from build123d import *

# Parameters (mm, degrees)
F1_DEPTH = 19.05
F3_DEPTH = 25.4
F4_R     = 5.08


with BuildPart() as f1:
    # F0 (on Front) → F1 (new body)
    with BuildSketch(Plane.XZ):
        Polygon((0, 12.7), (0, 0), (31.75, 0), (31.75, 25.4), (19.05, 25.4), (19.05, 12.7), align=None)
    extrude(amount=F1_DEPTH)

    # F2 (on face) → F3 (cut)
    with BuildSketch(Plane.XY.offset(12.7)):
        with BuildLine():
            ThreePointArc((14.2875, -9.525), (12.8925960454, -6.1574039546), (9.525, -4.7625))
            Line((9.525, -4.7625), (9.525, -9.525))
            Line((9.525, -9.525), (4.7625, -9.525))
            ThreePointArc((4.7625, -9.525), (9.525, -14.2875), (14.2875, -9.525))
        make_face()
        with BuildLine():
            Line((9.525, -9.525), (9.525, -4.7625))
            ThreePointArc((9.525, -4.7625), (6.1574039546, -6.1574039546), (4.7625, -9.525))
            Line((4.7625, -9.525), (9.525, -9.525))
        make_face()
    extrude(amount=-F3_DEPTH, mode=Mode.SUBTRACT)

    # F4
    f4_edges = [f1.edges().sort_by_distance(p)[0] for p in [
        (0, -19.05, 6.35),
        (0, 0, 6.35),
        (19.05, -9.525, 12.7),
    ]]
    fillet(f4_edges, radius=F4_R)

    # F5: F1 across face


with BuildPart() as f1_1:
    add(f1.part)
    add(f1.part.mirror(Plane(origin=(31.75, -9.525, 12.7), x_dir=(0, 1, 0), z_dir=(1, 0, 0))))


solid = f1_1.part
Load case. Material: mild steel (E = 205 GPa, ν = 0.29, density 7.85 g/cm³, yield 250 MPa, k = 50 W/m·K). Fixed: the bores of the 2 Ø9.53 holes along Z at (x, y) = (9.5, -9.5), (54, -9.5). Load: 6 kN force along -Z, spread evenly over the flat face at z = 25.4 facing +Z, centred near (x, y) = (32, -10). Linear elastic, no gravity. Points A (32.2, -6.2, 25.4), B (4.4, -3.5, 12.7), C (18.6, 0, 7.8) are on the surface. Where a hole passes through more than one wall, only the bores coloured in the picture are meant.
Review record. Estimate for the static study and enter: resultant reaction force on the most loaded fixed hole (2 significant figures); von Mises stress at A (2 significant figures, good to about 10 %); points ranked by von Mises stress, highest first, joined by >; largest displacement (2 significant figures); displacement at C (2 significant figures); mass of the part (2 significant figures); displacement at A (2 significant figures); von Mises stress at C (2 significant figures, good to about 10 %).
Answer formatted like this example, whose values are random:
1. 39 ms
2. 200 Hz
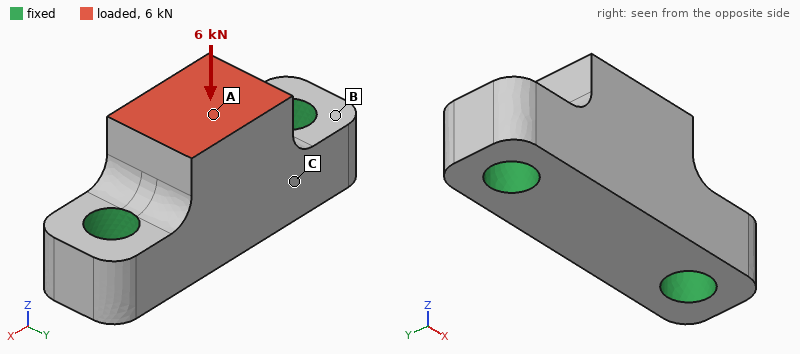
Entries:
1. 3.2 kN
2. 11 MPa
3. C > A > B
4. 2.9 µm
5. 1.4 µm
6. 150 g
7. 2.9 µm
8. 19 MPa
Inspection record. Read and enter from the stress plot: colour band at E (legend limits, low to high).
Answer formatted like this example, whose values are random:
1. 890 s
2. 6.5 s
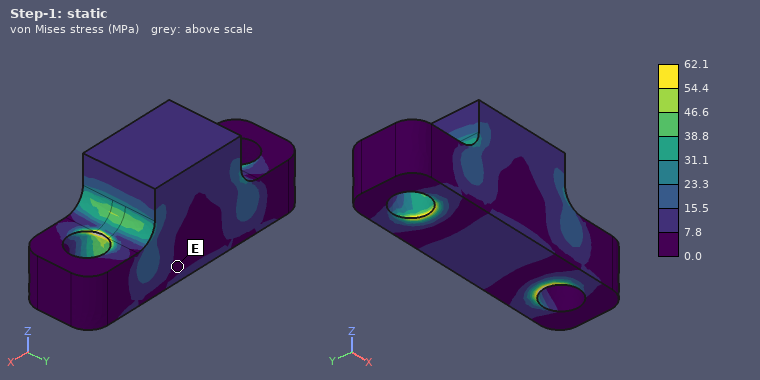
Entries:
1. 0.0 to 7.8 MPa
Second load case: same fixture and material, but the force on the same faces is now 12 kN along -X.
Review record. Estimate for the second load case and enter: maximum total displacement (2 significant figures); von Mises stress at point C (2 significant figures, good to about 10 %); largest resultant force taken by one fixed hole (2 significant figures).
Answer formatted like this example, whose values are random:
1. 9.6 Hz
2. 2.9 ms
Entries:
1. 12 µm
2. 29 MPa
3. 8.6 kN
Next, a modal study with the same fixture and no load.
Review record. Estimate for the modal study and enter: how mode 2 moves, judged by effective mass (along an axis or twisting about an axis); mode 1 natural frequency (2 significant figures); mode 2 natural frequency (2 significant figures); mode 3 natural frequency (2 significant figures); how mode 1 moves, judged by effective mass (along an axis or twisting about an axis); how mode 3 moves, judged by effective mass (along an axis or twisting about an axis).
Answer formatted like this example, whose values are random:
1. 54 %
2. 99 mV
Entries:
1. along Z
2. 16 kHz
3. 26 kHz
4. 31 kHz
5. along Y
6. along Y
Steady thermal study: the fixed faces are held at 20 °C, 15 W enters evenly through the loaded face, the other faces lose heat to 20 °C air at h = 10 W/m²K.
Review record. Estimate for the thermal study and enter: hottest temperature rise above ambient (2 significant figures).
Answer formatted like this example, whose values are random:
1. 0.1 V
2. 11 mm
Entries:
1. 15 K
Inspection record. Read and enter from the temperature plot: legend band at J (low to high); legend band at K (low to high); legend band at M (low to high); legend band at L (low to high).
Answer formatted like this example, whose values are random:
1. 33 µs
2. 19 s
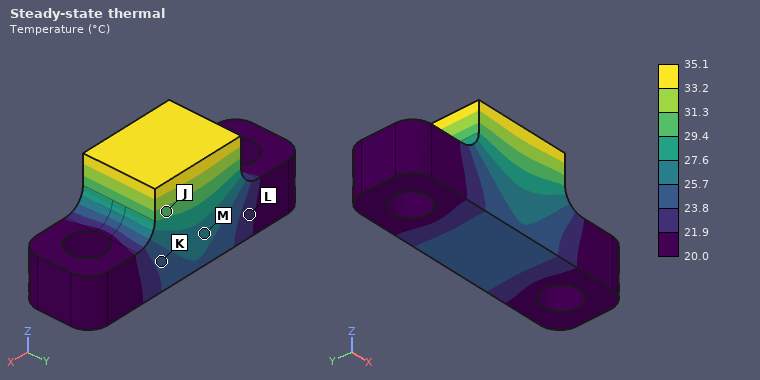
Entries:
1. 29.4 to 31.3 °C
2. 23.8 to 25.7 °C
3. 25.7 to 27.6 °C
4. 21.9 to 23.8 °C
